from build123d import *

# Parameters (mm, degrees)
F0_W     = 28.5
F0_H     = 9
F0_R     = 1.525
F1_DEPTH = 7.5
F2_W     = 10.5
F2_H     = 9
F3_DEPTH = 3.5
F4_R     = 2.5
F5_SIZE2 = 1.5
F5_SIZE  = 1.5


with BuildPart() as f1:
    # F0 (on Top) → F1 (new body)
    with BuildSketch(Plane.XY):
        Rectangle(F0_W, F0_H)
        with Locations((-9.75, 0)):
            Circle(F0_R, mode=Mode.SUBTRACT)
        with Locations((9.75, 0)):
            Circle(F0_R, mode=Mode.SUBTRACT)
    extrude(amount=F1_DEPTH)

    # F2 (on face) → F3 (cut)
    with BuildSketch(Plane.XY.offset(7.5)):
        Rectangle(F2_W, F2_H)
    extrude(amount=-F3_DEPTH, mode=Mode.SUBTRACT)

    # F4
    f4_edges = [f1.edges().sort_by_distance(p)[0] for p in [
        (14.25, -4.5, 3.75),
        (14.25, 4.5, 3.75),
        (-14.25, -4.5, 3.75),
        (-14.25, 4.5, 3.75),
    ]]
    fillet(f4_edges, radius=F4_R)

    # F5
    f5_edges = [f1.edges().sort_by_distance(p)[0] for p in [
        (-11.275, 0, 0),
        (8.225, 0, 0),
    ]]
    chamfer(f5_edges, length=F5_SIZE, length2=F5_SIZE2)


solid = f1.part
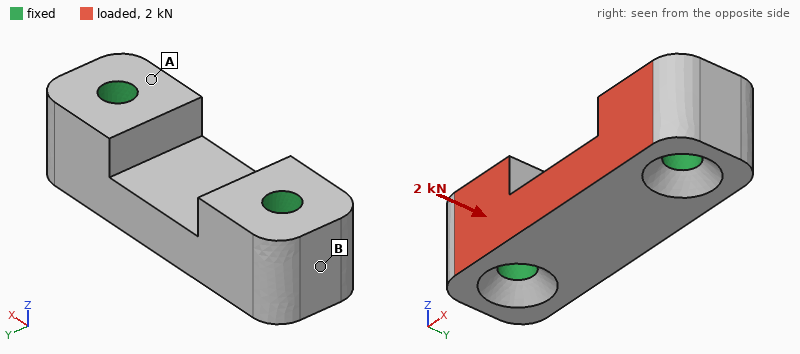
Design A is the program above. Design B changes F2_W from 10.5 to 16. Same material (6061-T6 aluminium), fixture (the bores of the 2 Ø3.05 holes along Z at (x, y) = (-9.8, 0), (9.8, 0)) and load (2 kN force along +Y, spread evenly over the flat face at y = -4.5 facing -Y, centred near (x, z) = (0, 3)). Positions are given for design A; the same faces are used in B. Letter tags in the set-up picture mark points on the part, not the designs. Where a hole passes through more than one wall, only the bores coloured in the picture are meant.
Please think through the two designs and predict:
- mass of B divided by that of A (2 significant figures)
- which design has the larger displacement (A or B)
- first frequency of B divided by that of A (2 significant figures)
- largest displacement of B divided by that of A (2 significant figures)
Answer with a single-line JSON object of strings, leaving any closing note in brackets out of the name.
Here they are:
{"mass of B divided by that of A": "0.88", "which design has the larger displacement": "B", "first frequency of B divided by that of A": "0.76", "largest displacement of B divided by that of A": "1.2"}
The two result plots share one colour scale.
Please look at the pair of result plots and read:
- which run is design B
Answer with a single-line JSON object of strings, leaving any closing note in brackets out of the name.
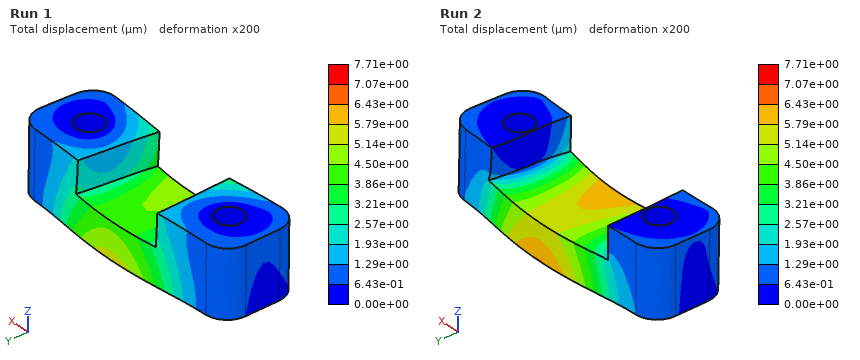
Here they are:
{"which run is design B": "Run 2"}
